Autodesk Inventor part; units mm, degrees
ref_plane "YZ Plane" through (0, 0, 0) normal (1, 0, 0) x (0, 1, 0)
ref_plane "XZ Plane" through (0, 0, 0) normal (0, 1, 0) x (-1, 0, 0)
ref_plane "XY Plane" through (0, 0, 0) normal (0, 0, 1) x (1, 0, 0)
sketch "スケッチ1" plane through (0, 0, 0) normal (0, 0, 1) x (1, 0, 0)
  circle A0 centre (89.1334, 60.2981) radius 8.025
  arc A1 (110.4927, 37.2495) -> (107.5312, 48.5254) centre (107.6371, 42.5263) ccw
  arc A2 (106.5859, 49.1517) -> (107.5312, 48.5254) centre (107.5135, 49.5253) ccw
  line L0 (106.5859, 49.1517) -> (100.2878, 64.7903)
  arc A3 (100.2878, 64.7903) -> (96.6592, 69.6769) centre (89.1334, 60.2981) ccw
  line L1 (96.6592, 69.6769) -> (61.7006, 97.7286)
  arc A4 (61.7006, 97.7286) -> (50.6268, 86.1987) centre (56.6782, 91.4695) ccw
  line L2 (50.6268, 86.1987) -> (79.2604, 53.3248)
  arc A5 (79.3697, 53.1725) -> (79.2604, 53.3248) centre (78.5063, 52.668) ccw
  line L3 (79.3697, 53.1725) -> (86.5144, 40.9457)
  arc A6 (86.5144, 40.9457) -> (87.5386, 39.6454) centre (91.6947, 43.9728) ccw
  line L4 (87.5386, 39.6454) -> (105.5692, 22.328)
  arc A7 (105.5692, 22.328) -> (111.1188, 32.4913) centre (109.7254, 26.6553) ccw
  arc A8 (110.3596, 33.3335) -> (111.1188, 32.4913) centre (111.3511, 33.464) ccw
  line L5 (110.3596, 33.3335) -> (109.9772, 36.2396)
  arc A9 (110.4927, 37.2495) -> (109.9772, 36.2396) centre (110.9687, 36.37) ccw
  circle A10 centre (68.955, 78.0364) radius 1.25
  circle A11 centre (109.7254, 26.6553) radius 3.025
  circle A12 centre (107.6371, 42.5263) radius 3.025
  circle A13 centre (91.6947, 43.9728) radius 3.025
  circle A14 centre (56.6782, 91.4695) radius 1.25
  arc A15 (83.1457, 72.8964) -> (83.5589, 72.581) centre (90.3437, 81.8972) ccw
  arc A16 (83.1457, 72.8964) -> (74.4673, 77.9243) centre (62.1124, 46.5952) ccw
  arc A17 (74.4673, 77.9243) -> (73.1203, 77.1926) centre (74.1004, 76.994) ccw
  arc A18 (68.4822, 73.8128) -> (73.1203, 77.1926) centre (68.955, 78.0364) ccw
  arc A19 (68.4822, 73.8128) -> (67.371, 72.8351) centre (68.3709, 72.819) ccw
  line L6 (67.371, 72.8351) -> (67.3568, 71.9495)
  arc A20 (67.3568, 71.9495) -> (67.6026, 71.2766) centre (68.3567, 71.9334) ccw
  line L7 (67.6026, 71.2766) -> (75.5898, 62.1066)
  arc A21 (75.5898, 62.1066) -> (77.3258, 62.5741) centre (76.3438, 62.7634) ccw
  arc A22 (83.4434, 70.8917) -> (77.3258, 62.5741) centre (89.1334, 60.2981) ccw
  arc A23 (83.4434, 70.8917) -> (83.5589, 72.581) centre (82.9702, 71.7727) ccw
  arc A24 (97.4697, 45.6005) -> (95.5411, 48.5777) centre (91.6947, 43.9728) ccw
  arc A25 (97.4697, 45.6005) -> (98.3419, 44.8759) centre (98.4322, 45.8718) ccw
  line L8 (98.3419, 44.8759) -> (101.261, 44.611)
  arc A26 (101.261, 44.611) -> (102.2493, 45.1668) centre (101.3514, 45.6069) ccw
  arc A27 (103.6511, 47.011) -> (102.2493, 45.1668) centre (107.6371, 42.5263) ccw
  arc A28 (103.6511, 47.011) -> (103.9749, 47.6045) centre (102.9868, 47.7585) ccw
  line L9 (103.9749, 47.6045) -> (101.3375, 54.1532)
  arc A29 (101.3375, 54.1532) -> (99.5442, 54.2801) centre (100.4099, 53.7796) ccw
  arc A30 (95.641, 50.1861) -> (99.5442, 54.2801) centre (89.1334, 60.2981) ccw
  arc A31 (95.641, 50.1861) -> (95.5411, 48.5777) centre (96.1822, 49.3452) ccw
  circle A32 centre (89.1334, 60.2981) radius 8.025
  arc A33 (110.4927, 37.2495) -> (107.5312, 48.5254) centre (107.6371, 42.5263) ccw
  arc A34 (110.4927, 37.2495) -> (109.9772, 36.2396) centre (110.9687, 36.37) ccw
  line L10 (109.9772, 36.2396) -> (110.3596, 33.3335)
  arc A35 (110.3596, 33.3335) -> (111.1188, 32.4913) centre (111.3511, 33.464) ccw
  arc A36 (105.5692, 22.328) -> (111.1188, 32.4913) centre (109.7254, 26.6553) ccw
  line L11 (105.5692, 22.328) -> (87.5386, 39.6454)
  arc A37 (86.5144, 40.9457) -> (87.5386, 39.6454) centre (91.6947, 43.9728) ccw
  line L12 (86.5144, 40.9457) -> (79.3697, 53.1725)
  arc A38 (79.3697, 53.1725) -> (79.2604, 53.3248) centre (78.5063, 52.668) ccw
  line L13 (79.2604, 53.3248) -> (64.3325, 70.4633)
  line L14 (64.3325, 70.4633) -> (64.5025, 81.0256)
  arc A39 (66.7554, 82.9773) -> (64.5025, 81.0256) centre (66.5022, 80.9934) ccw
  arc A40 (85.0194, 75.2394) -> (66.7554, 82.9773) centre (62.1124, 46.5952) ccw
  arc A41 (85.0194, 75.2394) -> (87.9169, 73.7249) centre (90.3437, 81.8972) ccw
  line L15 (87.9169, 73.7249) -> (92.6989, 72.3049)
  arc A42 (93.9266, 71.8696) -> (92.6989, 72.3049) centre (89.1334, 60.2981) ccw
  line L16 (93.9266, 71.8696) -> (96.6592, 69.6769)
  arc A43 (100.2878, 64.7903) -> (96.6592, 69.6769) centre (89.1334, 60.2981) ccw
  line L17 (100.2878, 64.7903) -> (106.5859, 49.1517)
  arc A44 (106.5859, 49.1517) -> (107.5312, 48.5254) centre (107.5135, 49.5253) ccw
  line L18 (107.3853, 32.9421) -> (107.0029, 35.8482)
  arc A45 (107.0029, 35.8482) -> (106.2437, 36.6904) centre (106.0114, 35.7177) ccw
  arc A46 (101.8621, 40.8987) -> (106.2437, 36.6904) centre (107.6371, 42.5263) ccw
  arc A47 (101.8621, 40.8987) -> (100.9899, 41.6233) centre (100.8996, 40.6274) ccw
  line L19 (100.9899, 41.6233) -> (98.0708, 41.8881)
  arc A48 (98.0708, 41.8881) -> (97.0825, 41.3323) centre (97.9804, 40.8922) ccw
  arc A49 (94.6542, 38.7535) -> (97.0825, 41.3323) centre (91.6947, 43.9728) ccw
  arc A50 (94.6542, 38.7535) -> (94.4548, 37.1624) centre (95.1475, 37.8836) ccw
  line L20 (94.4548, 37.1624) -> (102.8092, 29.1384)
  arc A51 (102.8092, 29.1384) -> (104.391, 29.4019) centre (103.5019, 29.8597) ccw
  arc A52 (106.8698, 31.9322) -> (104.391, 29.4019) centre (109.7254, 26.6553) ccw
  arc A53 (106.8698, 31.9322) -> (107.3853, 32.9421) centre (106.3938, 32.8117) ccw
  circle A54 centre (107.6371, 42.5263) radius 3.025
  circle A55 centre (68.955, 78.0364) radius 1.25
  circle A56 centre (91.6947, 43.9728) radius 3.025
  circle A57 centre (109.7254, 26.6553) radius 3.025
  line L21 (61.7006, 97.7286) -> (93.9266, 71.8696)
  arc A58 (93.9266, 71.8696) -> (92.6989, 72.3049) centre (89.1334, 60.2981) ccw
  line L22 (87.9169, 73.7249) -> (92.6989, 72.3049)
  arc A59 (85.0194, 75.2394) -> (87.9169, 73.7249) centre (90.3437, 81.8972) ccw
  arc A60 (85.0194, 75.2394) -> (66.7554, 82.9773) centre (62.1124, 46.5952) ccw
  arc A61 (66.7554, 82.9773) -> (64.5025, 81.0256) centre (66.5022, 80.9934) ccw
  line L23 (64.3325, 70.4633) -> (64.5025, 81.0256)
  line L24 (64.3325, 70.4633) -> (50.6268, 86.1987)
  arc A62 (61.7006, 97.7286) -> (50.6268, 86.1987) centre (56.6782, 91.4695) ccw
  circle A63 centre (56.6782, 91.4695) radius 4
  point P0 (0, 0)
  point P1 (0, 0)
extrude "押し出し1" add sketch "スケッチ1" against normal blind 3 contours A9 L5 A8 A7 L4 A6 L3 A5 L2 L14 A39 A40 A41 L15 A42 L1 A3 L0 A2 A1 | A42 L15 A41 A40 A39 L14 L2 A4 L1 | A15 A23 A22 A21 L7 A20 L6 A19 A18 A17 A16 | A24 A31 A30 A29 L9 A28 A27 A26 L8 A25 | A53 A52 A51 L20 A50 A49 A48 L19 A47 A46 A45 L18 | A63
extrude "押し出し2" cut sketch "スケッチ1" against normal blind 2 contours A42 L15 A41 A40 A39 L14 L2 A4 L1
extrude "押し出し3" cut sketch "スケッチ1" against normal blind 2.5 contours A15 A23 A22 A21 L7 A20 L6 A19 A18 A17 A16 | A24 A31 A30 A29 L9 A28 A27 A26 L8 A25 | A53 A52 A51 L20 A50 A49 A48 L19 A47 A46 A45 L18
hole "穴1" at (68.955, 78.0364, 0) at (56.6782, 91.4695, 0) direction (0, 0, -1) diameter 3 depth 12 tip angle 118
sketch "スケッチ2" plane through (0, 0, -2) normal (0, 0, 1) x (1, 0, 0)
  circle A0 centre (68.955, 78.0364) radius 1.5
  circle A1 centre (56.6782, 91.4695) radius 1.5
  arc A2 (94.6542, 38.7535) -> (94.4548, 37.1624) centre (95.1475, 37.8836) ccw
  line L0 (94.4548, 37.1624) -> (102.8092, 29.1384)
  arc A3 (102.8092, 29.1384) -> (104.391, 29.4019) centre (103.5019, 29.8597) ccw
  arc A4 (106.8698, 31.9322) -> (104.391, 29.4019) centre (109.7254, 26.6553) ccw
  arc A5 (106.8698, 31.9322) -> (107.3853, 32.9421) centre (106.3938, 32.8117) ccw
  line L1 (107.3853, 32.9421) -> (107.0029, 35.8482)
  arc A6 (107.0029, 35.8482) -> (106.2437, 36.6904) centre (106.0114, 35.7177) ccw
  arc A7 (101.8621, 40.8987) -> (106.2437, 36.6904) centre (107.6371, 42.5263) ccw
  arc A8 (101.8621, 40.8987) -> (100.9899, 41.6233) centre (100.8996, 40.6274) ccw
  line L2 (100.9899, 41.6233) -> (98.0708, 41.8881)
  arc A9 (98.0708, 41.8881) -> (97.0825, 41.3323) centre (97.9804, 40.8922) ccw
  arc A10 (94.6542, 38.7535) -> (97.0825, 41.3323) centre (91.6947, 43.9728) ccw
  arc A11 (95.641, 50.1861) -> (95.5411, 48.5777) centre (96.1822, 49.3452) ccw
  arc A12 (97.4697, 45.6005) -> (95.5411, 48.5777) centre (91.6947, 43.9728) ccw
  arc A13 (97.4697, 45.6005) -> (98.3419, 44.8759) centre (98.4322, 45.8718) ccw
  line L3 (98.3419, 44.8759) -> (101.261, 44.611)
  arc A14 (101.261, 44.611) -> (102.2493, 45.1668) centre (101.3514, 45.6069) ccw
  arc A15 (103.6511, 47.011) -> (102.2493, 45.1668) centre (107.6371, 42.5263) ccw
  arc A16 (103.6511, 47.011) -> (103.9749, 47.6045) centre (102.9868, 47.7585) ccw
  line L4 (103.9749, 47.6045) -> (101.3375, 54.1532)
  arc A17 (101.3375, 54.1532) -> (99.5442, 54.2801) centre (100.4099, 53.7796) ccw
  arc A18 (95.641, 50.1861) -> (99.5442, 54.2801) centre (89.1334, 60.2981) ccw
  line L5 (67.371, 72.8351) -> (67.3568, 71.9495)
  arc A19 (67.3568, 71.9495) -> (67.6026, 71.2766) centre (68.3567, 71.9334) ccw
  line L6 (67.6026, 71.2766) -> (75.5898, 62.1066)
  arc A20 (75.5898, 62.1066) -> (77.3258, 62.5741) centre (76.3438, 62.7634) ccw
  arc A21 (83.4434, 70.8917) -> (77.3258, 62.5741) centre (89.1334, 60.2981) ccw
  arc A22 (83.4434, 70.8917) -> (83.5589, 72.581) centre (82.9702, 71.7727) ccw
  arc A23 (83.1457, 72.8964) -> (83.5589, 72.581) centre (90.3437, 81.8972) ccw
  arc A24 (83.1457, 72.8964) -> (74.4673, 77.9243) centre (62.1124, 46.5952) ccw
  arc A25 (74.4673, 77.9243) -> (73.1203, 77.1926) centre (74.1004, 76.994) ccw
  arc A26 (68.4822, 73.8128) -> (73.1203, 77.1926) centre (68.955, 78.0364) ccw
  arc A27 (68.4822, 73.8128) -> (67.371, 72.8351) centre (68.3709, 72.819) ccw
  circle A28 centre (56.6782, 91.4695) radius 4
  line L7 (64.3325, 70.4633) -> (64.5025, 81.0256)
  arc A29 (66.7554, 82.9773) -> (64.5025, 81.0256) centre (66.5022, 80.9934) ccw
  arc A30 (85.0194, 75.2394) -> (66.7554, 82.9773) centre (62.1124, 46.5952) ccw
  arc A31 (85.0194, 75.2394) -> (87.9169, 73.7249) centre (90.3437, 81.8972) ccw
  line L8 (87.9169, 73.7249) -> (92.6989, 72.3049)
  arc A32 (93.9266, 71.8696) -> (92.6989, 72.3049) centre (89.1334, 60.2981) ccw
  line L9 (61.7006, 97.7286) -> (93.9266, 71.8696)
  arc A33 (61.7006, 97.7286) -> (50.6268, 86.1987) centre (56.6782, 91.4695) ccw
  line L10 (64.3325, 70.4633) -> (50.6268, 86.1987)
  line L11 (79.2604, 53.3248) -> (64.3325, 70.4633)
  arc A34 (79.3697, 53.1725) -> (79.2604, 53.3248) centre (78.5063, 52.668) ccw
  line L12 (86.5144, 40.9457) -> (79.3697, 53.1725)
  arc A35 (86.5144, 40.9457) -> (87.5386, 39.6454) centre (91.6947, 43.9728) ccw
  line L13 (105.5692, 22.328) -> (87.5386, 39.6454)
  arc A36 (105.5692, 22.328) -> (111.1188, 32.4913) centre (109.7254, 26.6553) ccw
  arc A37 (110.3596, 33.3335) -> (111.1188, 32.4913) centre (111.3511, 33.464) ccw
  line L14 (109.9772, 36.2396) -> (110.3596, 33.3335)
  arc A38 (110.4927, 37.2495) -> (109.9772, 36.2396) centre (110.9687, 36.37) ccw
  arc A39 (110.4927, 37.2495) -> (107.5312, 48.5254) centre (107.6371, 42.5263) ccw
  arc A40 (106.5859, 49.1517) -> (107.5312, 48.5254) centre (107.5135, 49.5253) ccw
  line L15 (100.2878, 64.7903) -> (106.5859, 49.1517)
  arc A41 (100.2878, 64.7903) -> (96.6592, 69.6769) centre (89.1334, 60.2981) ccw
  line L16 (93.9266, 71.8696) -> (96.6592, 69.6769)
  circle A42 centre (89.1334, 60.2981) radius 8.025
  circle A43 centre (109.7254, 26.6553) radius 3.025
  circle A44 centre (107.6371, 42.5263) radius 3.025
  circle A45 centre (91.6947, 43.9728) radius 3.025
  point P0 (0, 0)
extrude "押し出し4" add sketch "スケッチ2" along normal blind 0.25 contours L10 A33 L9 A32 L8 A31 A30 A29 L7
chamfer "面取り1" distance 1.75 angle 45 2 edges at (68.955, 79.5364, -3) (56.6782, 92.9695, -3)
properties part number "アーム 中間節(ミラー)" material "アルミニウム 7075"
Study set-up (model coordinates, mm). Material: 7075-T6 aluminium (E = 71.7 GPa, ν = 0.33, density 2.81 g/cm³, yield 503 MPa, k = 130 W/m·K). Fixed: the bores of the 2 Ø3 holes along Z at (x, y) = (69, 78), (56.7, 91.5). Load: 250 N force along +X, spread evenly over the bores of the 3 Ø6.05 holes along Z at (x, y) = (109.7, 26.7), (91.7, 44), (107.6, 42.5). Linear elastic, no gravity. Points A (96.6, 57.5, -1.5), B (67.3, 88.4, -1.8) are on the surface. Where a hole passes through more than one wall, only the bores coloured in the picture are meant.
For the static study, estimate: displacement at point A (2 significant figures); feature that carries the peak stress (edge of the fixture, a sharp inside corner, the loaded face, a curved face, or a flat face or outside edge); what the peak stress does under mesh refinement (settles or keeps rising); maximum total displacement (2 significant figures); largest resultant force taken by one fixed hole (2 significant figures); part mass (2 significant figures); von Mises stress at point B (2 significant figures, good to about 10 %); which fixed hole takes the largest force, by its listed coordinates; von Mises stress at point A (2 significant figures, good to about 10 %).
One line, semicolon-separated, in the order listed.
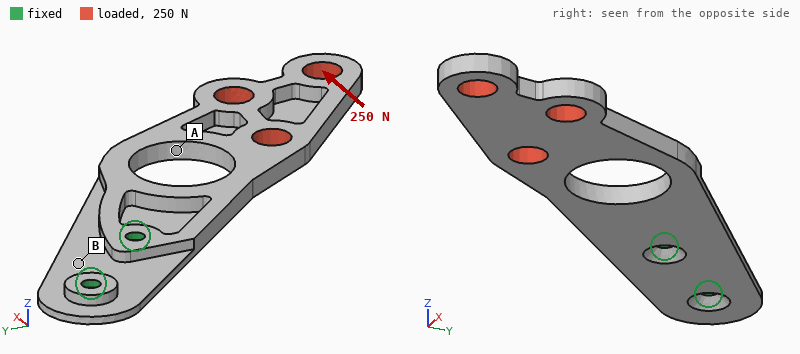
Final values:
0.18 mm; edge of the fixture; keeps rising; 0.38 mm; 620 N; 9.0 g; 55 MPa; (69, 78); 15 MPa
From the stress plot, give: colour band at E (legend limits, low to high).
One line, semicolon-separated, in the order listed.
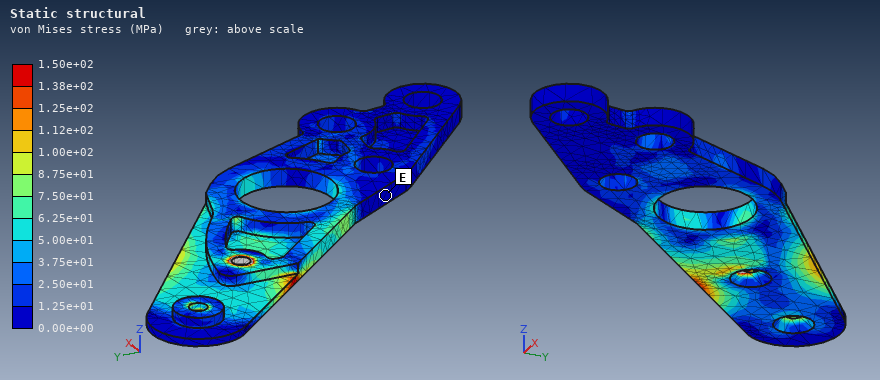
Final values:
0.00e+00 to 1.25e+01 MPa
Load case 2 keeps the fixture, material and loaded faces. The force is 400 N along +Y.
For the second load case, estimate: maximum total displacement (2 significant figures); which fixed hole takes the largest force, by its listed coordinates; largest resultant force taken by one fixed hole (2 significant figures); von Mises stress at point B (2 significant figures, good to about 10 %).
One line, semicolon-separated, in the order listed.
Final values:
0.59 mm; (69, 78); 840 N; 78 MPa
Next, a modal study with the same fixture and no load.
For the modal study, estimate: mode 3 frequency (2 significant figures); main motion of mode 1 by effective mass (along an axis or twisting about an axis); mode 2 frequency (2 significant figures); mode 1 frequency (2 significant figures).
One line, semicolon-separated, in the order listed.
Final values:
2200 Hz; along Z; 2000 Hz; 420 Hz
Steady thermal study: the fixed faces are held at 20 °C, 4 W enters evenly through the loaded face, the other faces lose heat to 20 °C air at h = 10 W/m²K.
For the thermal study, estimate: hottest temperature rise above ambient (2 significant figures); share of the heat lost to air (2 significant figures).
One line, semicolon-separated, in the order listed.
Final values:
48 K; 22 %
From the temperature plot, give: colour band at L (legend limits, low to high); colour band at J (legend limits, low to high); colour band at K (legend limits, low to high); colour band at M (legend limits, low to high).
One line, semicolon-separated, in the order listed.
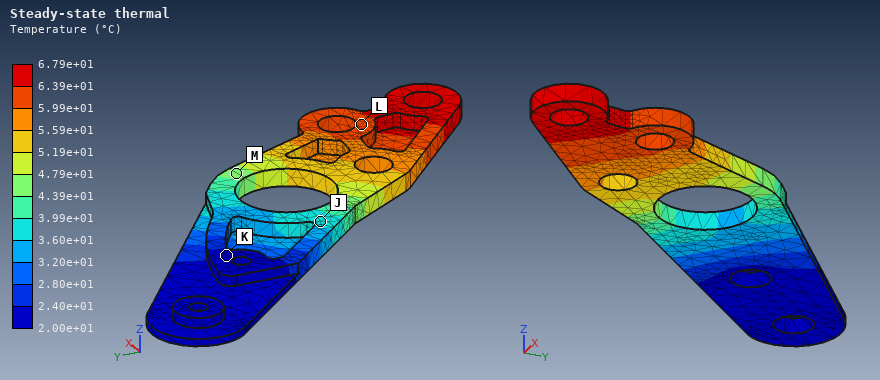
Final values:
5.99e+01 to 6.39e+01 °C; 3.60e+01 to 3.99e+01 °C; 2.00e+01 to 2.40e+01 °C; 4.39e+01 to 4.79e+01 °C
